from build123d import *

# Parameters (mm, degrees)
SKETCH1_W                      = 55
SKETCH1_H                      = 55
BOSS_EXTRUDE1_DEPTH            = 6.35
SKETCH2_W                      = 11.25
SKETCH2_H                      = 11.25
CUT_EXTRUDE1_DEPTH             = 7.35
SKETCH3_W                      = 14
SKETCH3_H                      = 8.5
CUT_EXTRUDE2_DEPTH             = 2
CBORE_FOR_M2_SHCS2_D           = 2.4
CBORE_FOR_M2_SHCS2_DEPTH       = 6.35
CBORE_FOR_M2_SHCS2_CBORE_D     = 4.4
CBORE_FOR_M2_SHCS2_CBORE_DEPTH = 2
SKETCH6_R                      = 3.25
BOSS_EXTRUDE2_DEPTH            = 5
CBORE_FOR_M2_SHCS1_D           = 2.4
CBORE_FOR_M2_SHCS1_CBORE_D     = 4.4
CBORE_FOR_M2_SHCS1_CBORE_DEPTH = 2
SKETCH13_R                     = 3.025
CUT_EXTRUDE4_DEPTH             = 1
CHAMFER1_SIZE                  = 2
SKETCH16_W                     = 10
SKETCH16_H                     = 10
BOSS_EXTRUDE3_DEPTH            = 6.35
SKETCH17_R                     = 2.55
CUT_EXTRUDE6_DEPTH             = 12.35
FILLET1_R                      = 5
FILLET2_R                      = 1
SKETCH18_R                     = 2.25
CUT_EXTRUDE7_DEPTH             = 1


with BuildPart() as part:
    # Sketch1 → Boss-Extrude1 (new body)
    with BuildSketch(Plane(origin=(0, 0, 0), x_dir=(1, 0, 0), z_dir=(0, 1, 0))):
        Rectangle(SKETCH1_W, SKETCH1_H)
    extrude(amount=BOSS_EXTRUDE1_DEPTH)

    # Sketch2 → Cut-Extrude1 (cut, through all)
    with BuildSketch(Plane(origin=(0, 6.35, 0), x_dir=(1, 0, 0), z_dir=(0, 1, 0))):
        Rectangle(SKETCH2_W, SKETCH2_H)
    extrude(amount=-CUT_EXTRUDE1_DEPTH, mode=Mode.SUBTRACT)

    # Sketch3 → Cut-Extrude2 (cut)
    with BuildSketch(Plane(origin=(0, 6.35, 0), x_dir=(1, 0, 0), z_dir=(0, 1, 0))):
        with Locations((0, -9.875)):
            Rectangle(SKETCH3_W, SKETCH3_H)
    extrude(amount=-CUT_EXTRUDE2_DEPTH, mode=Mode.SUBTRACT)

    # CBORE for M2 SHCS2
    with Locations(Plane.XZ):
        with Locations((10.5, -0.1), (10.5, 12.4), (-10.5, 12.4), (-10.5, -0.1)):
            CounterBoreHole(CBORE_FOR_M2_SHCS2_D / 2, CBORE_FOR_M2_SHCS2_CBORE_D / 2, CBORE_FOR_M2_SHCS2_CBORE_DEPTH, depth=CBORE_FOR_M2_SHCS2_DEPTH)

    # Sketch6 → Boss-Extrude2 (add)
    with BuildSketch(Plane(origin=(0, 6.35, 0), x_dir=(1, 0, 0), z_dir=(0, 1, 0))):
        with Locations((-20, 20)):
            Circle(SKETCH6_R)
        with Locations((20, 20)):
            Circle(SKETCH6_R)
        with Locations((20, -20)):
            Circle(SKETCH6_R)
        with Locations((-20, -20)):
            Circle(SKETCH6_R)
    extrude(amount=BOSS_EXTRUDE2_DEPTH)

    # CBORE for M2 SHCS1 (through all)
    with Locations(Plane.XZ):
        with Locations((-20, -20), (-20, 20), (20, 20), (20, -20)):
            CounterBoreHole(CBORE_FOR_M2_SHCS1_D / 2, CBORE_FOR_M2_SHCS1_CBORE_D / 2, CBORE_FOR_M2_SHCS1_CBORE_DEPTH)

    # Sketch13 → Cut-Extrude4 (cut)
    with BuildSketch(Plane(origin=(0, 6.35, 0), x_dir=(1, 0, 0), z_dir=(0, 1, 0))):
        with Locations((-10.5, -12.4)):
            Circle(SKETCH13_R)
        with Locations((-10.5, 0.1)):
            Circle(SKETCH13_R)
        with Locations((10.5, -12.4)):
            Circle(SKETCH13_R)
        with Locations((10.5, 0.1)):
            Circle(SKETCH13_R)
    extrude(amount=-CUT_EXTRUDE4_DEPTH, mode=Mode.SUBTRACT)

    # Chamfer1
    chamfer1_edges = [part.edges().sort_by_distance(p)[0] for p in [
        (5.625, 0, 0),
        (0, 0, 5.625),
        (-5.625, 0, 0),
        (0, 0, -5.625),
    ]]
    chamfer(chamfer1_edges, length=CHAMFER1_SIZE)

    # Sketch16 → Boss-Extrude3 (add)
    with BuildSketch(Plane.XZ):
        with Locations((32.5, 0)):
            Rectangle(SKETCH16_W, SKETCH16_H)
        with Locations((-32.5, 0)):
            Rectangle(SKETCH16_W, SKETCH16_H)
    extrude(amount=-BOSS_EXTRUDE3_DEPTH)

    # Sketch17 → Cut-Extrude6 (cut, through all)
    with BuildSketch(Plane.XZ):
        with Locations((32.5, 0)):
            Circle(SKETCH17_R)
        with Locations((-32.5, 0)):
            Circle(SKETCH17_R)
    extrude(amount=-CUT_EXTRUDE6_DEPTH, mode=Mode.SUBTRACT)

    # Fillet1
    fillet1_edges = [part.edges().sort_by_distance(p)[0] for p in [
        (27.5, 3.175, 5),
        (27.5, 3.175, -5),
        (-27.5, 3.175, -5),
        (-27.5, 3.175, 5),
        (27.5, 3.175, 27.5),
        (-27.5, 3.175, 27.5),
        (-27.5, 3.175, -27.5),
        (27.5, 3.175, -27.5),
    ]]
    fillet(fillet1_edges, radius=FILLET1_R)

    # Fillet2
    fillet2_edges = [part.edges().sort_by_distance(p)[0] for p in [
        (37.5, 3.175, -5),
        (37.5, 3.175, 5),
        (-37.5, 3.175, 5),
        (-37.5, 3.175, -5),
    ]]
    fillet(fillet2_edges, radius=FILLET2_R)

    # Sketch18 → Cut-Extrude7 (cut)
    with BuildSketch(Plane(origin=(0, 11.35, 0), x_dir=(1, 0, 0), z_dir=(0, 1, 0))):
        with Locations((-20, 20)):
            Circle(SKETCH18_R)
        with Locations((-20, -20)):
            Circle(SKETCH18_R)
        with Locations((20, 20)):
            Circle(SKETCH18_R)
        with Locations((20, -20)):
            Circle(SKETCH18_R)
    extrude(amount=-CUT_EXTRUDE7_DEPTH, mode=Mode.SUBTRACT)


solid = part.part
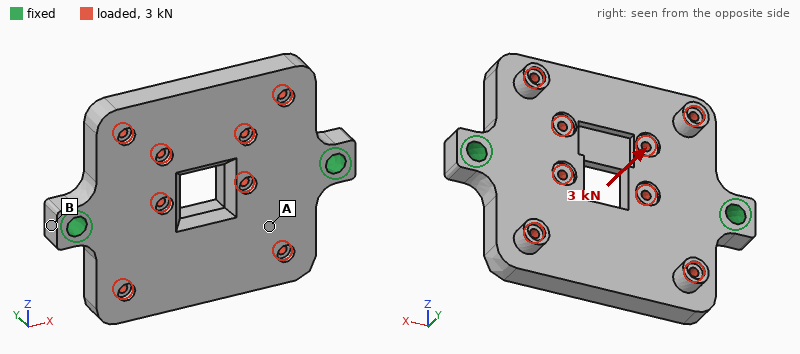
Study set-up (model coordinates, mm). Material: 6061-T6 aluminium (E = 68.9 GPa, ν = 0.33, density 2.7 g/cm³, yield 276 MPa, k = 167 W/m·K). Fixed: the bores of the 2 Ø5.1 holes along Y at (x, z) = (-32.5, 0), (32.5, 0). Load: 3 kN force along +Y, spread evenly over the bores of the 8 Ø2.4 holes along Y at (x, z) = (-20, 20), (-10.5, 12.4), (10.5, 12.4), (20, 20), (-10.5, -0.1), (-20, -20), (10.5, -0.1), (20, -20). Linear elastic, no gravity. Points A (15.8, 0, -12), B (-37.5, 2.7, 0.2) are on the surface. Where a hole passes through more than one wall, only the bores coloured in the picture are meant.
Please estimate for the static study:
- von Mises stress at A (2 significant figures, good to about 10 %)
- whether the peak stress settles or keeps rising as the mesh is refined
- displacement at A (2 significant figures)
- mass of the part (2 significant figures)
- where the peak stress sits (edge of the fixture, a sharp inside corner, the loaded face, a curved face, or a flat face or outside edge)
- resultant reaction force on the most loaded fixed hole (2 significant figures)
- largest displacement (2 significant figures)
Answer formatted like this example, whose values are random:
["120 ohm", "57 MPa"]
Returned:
["39 MPa", "keeps rising", "0.050 mm", "52 g", "edge of the fixture", "1.5 kN", "0.16 mm"]
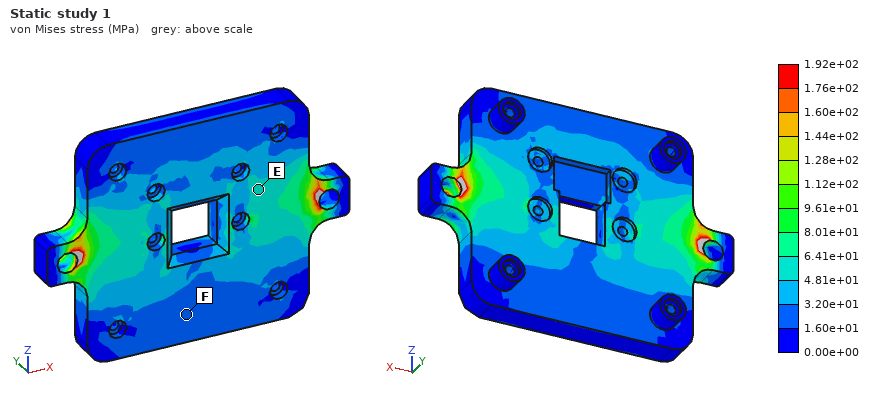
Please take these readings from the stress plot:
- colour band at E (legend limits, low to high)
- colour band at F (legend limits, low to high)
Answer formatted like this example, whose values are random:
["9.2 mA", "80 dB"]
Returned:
["4.81e+01 to 6.41e+01 MPa", "1.60e+01 to 3.20e+01 MPa"]
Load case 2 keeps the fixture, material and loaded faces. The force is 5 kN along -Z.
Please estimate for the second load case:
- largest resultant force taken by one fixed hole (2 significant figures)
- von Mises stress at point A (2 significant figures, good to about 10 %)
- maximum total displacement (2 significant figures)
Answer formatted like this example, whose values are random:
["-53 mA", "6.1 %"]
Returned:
["2.5 kN", "18 MPa", "83 µm"]
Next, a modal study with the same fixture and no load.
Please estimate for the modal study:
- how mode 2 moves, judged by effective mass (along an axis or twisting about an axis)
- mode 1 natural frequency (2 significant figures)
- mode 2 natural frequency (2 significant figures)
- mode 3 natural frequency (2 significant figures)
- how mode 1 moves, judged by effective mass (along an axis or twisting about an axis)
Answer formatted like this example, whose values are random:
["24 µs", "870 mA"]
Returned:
["along Y", "3000 Hz", "4300 Hz", "7800 Hz", "twisting about X"]
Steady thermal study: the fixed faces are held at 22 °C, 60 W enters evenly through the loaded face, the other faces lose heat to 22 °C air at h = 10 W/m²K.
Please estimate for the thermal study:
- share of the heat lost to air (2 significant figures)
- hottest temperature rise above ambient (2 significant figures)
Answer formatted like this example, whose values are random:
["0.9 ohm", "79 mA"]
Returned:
["3.2 %", "32 K"]
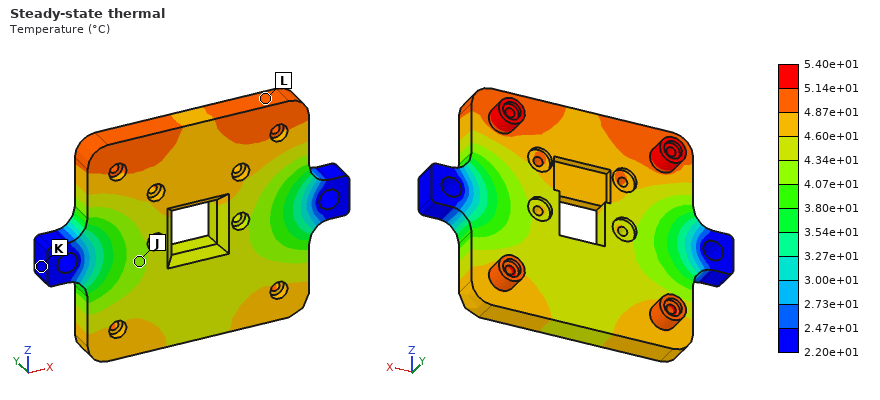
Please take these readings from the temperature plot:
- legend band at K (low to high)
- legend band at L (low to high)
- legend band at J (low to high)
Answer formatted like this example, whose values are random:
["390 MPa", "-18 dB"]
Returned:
["2.20e+01 to 2.47e+01 °C", "4.87e+01 to 5.14e+01 °C", "4.07e+01 to 4.34e+01 °C"]
